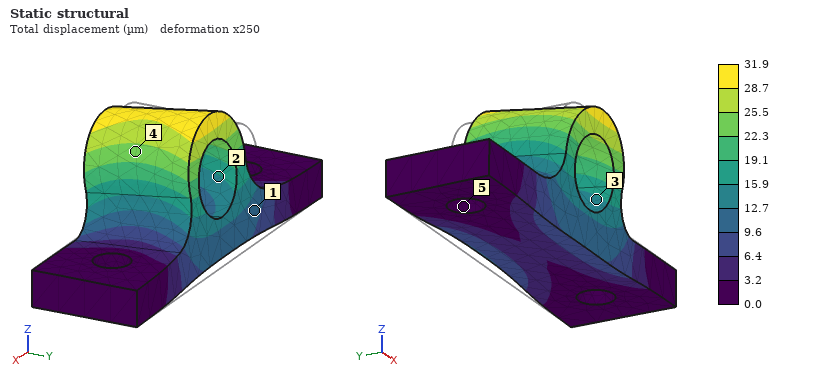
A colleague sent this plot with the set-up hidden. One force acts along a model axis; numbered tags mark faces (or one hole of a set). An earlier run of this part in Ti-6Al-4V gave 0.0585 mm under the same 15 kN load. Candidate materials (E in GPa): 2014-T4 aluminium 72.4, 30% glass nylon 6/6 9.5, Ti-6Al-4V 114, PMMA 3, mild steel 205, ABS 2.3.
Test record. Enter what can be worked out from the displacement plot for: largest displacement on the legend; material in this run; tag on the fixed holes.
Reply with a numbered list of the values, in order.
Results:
1. 31.9 µm
2. mild steel
3. 5
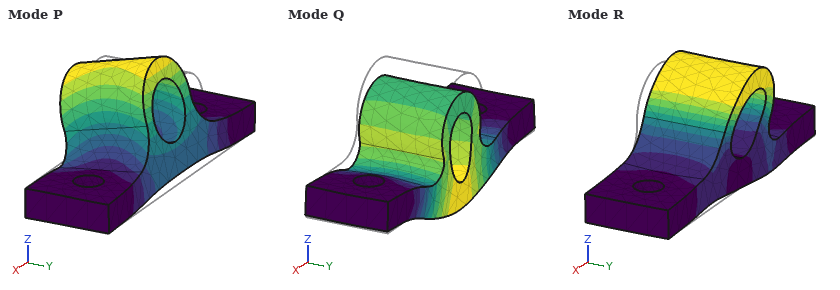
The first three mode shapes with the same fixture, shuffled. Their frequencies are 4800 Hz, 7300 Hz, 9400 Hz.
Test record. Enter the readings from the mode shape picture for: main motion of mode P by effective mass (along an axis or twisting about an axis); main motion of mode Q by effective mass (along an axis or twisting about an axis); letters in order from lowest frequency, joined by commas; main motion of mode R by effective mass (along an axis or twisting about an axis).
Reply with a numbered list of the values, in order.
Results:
1. along Y
2. along Z
3. P, Q, R
4. along X
